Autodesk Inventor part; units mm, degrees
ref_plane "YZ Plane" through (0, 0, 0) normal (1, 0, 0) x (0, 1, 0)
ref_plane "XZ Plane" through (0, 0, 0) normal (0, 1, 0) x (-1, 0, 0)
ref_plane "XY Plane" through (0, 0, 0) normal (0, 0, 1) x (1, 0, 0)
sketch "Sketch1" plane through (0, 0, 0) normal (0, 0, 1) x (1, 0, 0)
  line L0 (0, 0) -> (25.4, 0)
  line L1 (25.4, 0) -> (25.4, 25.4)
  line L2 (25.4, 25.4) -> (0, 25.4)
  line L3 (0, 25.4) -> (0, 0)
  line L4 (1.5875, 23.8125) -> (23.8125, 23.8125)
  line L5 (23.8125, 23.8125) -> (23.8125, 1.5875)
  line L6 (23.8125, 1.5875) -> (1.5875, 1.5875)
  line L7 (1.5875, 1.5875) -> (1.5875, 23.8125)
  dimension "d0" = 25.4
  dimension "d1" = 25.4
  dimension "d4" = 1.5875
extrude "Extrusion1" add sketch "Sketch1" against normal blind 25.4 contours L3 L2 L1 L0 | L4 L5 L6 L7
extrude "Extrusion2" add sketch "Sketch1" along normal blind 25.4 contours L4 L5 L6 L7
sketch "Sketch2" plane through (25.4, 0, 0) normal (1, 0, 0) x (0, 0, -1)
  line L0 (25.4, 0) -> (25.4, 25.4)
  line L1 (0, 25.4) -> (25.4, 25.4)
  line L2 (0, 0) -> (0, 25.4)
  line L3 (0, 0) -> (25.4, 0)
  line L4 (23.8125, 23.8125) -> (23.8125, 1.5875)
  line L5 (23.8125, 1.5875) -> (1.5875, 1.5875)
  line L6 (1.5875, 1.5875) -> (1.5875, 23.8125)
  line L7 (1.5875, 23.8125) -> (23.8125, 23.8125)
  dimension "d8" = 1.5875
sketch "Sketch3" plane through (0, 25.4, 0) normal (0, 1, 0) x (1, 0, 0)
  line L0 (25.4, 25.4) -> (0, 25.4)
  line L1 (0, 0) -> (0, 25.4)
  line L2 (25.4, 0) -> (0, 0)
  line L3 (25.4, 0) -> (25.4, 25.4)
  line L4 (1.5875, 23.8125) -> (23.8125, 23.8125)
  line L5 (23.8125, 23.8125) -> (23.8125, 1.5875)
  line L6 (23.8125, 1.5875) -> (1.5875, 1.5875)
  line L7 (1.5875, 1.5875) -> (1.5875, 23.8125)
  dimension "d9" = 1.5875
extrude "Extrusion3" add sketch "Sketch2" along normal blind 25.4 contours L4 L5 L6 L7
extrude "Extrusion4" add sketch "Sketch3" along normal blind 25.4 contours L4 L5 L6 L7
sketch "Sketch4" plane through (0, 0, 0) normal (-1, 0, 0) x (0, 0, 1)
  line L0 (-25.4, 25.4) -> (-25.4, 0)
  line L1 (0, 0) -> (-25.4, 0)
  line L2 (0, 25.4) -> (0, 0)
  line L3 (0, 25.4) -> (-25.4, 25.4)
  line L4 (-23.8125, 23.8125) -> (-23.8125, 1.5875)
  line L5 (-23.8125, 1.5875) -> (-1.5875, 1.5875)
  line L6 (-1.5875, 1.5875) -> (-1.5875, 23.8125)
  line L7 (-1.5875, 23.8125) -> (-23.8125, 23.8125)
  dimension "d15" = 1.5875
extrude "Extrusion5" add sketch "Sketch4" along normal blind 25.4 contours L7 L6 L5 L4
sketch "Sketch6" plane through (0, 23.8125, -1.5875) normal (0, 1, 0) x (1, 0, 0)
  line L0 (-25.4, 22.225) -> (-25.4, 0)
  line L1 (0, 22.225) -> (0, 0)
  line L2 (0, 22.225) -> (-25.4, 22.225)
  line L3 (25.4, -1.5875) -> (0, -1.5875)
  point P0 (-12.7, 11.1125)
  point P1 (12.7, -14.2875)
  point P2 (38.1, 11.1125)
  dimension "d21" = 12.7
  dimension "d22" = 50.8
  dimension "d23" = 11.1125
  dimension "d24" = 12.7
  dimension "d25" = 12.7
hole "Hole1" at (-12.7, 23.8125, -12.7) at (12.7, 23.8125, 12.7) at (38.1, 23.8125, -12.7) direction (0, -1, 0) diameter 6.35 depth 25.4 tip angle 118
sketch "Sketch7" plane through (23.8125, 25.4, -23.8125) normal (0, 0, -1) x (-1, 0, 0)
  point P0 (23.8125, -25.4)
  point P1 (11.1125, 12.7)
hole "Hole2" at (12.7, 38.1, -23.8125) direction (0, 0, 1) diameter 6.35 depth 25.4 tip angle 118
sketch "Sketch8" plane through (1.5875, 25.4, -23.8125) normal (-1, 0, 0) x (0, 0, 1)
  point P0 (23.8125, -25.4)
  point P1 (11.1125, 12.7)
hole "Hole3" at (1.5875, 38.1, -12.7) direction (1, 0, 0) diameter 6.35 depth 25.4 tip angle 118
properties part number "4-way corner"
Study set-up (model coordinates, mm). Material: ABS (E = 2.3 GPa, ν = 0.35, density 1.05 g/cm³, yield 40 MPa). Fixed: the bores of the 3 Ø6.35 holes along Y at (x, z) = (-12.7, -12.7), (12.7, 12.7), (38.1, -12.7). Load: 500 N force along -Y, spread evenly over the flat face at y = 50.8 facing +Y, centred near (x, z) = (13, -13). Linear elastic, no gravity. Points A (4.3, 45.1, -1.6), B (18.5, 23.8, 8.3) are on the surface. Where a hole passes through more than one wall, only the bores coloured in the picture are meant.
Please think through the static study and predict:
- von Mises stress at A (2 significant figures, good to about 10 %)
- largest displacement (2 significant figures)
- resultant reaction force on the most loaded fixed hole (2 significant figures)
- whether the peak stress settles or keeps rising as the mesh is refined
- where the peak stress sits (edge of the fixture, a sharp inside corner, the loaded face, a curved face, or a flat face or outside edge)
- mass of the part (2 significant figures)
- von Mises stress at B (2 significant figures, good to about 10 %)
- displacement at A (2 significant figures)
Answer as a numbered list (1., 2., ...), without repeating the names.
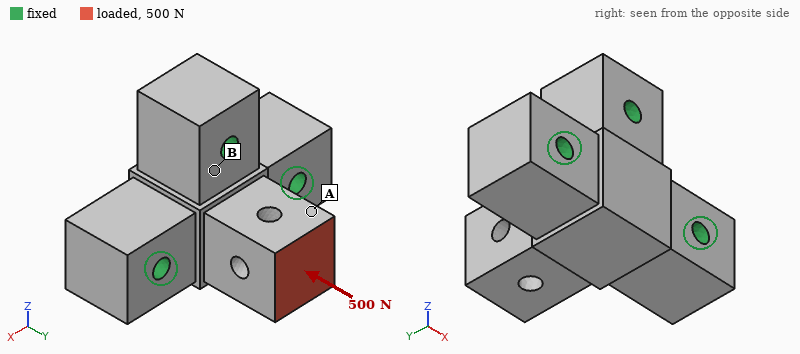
1. 1.2 MPa
2. 36 µm
3. 200 N
4. keeps rising
5. a sharp inside corner
6. 66 g
7. 0.46 MPa
8. 22 µm
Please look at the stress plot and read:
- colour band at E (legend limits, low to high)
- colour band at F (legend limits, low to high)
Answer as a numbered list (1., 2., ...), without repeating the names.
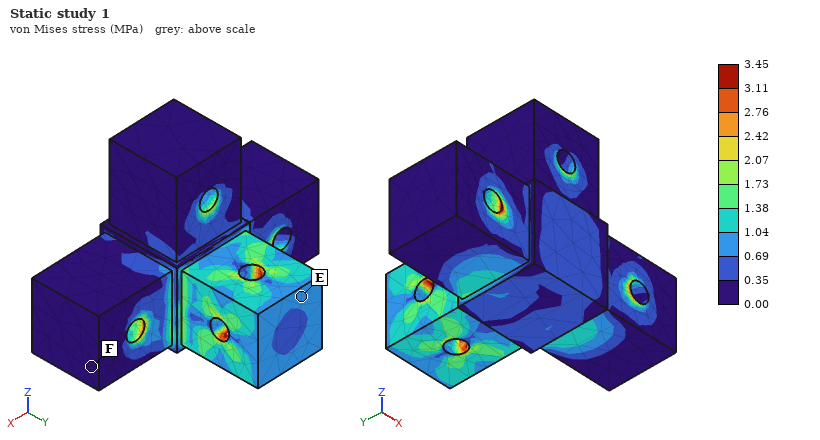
1. 0.69 to 1.04 MPa
2. 0.00 to 0.35 MPa
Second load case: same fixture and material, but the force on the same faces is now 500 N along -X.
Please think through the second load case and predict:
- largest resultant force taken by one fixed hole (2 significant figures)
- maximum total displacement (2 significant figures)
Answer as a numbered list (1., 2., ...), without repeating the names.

1. 450 N
2. 0.21 mm
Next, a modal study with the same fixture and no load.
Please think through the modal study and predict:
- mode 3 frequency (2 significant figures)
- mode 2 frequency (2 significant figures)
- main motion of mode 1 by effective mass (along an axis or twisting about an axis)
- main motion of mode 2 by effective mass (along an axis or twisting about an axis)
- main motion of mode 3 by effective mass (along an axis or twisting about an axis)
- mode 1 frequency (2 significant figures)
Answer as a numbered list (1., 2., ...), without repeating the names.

1. 6100 Hz
2. 3800 Hz
3. along Z
4. along X
5. along Y
6. 3200 Hz
